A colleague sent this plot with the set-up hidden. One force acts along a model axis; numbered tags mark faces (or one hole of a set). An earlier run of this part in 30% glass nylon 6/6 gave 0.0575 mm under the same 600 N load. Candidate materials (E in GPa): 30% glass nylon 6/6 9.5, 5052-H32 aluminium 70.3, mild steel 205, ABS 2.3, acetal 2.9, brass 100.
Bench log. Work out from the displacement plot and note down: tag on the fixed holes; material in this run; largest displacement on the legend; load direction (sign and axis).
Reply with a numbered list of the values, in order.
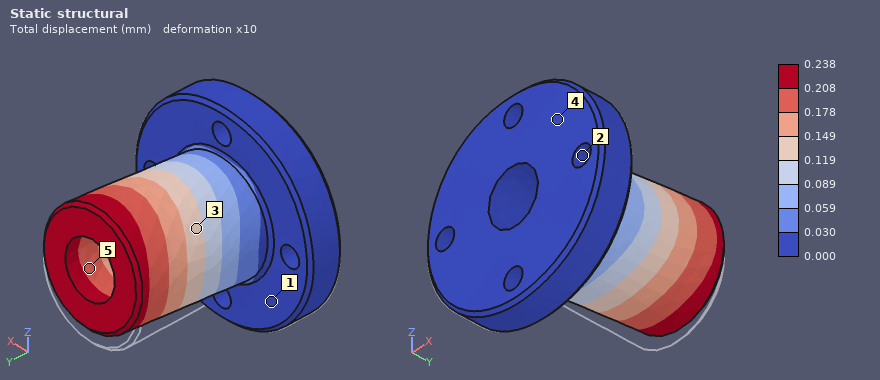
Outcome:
1. 2
2. ABS
3. 0.238 mm
4. +Z
